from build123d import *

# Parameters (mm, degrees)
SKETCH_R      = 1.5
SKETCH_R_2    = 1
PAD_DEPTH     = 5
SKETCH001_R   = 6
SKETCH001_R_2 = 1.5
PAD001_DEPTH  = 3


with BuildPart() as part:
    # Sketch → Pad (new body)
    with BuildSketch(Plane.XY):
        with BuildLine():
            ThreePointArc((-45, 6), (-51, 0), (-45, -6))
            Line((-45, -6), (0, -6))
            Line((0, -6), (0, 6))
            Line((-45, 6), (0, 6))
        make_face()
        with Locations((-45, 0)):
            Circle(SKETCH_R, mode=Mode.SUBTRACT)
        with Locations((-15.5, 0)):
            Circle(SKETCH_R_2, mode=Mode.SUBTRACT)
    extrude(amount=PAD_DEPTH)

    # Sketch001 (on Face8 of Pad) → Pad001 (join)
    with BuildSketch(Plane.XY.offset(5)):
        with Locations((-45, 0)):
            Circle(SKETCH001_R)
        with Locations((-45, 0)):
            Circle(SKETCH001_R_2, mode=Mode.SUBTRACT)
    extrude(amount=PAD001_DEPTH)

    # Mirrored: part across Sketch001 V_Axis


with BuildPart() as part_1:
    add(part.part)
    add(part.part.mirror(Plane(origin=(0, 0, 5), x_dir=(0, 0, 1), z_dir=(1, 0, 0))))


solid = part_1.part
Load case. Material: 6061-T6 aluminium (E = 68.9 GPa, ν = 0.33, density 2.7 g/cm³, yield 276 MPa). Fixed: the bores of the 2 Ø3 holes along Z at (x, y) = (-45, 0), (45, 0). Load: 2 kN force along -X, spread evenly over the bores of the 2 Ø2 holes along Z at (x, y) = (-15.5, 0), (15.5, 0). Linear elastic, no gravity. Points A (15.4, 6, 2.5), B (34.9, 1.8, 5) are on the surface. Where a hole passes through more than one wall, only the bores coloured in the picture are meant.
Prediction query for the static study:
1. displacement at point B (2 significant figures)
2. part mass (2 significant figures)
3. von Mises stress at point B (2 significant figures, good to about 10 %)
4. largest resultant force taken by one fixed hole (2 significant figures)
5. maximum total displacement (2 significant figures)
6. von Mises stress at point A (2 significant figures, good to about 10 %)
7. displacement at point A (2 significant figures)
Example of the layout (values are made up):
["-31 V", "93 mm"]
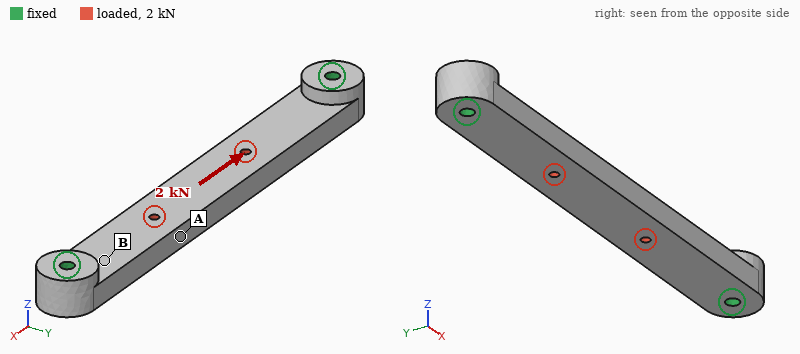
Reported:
["2.6 µm", "18 g", "19 MPa", "1.0 kN", "9.0 µm", "8.2 MPa", "6.9 µm"]
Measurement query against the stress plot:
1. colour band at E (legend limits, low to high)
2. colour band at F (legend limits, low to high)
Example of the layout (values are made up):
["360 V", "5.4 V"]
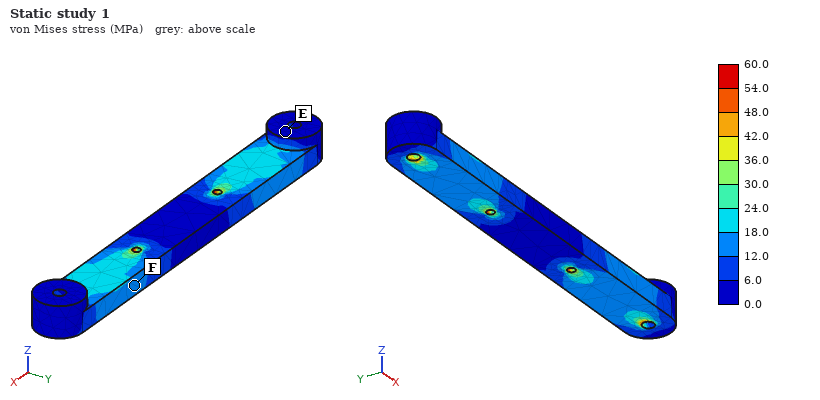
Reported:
["0.0 to 6.0 MPa", "12.0 to 18.0 MPa"]
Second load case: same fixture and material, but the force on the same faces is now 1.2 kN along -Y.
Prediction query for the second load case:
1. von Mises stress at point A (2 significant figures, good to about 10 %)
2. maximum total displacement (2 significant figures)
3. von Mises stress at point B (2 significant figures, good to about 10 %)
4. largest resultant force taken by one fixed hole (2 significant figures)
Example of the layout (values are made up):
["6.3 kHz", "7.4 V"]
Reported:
["63 MPa", "0.11 mm", "28 MPa", "600 N"]
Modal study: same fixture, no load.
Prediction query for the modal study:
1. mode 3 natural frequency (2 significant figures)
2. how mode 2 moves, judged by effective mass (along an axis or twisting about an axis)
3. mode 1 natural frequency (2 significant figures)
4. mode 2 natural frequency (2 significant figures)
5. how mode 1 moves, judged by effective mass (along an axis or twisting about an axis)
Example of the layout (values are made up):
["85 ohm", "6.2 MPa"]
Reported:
["9300 Hz", "along Y", "3500 Hz", "5800 Hz", "along Z"]
